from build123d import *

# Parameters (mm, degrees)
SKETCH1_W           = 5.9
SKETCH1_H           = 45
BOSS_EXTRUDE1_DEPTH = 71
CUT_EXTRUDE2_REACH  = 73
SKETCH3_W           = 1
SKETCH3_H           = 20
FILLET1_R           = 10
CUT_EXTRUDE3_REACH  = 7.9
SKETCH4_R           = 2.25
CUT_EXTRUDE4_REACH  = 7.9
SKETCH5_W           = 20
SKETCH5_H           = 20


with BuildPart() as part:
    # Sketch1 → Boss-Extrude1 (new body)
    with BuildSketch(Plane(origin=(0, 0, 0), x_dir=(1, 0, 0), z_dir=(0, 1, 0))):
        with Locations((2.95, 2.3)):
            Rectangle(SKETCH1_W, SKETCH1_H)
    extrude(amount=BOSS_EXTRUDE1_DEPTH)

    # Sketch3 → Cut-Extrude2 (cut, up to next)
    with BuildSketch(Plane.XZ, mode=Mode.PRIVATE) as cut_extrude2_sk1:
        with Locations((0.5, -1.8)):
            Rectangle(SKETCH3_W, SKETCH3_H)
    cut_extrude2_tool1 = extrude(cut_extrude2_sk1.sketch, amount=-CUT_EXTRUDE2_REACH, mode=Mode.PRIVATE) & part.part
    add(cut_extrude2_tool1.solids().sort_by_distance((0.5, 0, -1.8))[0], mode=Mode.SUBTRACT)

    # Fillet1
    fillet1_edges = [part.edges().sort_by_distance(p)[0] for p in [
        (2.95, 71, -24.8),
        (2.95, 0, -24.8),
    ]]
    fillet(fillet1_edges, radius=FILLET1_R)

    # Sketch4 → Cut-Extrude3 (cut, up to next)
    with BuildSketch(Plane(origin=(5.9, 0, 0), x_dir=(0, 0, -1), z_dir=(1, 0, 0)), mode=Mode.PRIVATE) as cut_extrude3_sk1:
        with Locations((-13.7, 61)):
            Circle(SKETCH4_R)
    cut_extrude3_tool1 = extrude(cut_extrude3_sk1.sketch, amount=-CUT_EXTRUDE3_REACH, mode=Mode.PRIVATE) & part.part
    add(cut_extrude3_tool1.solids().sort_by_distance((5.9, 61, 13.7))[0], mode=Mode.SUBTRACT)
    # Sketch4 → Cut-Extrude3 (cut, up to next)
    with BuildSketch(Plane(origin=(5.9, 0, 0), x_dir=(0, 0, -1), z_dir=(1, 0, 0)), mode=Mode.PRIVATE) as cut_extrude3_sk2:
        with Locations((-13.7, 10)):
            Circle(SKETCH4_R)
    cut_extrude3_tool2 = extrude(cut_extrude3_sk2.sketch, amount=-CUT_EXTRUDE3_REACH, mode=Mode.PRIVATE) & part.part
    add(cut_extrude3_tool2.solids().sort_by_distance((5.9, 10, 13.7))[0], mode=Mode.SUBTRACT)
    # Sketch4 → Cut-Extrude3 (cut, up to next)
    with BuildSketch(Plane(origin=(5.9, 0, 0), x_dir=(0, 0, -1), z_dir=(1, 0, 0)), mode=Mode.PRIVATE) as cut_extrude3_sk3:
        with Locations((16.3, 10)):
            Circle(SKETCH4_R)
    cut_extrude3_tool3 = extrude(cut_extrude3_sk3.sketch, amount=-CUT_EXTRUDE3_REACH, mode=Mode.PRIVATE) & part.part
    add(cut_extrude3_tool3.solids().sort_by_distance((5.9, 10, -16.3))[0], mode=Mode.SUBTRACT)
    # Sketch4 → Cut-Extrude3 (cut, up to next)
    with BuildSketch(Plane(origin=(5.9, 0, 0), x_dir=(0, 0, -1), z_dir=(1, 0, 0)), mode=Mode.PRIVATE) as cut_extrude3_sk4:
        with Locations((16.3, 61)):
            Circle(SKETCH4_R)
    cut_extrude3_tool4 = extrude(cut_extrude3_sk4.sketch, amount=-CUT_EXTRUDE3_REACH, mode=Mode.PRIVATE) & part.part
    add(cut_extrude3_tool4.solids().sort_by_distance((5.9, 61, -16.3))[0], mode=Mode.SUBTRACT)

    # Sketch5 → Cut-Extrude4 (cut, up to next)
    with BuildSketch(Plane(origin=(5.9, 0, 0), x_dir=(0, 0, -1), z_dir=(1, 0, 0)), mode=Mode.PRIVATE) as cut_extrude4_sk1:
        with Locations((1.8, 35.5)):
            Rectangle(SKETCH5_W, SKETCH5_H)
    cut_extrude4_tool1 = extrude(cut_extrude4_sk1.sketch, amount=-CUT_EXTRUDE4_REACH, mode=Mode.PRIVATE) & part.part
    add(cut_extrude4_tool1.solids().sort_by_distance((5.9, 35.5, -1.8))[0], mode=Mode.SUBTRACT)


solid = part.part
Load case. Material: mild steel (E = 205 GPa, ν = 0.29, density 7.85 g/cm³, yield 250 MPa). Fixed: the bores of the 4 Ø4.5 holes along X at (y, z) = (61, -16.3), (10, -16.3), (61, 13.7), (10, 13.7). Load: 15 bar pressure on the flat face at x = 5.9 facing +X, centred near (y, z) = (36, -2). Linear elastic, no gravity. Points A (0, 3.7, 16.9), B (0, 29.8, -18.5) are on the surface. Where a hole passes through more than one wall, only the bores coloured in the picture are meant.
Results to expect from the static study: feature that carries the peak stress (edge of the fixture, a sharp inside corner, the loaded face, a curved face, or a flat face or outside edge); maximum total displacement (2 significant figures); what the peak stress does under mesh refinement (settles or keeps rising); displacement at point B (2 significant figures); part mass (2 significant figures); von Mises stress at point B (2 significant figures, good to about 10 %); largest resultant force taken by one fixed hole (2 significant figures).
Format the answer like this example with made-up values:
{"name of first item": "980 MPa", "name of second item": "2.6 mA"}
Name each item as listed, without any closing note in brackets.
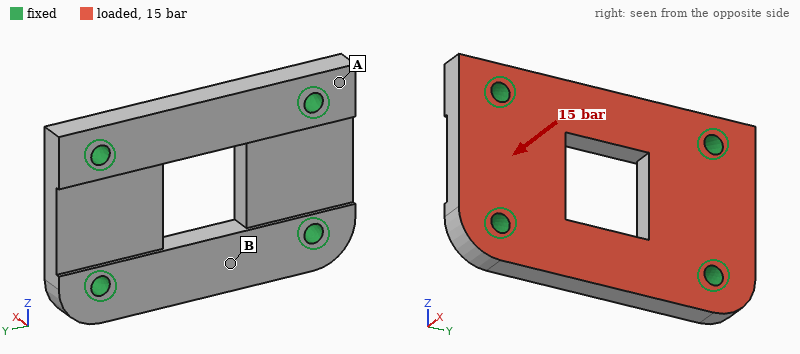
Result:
{"feature that carries the peak stress": "edge of the fixture", "maximum total displacement": "8.8 µm", "what the peak stress does under mesh refinement": "keeps rising", "displacement at point B": "7.5 µm", "part mass": "120 g", "von Mises stress at point B": "23 MPa", "largest resultant force taken by one fixed hole": "1.0 kN"}
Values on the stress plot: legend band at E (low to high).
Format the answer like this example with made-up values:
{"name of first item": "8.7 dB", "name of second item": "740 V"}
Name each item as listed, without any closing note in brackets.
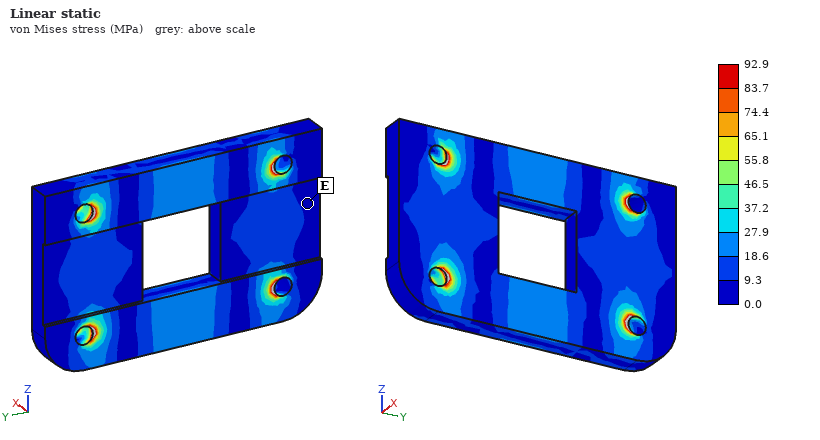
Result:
{"legend band at E": "0.0 to 9.3 MPa"}
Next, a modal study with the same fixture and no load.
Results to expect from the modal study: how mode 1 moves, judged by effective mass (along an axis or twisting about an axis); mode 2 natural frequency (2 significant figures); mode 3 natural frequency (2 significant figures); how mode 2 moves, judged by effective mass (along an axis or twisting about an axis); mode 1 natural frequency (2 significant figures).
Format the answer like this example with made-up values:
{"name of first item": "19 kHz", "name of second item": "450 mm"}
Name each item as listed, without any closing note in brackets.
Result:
{"how mode 1 moves, judged by effective mass": "along X", "mode 2 natural frequency": "13 kHz", "mode 3 natural frequency": "20 kHz", "how mode 2 moves, judged by effective mass": "twisting about Y", "mode 1 natural frequency": "12 kHz"}
